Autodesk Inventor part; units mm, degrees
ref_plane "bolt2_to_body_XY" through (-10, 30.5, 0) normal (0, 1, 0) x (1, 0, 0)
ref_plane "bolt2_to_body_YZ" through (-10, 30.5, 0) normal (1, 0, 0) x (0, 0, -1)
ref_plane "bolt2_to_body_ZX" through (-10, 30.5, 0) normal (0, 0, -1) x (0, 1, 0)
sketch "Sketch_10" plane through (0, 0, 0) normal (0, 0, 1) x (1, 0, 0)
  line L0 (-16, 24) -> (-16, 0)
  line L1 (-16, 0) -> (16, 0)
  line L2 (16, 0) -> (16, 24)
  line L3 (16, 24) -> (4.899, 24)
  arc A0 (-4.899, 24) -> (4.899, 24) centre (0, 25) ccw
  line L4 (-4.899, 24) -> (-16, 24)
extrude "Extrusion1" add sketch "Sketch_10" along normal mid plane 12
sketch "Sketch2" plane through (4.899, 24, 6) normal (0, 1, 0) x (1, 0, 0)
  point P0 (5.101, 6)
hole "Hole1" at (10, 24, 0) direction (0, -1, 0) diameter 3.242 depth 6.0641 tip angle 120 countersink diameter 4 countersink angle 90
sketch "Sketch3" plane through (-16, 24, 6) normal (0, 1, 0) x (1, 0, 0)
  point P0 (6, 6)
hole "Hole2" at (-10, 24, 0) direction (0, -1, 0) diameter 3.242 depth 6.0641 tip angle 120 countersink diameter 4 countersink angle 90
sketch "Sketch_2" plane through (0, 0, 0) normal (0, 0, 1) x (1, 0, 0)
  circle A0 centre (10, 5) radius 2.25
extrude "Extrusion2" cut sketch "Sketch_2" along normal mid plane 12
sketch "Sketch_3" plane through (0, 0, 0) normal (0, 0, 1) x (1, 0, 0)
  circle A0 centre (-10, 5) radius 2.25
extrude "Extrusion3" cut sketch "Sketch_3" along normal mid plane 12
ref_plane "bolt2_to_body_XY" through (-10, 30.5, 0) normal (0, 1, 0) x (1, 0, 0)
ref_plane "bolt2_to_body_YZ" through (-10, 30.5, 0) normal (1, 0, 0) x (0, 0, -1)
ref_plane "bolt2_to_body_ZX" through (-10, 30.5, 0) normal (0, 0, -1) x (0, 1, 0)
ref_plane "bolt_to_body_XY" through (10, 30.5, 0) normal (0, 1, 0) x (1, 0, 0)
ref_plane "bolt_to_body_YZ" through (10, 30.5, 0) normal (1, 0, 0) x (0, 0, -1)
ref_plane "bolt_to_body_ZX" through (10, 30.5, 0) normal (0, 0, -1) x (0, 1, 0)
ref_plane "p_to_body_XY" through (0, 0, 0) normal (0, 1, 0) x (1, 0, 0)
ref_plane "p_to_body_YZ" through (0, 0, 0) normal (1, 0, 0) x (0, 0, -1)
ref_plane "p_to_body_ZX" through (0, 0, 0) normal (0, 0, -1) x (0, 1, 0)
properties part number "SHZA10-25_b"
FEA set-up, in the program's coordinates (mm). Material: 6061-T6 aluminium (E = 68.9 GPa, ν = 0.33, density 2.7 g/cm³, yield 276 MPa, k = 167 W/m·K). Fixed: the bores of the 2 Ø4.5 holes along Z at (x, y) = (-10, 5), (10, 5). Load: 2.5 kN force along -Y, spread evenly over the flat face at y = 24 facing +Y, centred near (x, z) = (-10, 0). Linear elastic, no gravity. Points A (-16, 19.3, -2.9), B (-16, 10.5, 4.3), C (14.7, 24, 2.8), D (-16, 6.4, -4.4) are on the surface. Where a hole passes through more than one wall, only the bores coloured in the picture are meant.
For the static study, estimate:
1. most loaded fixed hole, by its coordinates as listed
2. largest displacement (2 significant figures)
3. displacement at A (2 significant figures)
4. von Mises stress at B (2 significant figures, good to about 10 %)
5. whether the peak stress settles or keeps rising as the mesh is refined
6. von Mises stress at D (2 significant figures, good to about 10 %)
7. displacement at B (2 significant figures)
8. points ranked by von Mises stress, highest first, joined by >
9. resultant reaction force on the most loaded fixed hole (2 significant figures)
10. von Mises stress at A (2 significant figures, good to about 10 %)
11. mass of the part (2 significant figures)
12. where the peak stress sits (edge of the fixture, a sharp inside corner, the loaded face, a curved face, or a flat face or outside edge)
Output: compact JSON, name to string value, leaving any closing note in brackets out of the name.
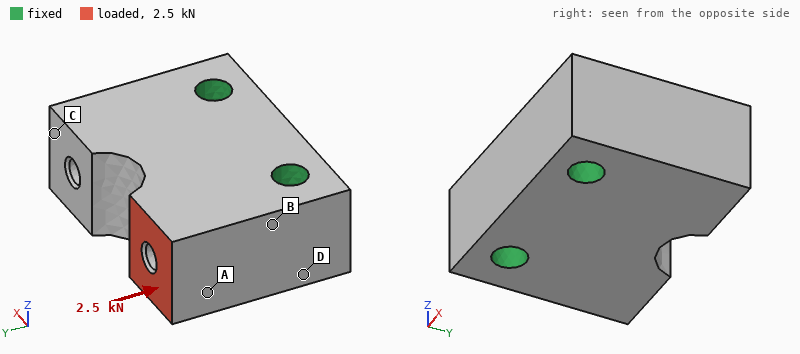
{"most loaded fixed hole, by its coordinates as listed": "(-10, 5)", "largest displacement": "7.5 µm", "displacement at A": "5.6 µm", "von Mises stress at B": "17 MPa", "whether the peak stress settles or keeps rising as the mesh is refined": "keeps rising", "von Mises stress at D": "10 MPa", "displacement at B": "2.5 µm", "points ranked by von Mises stress, highest first, joined by >": "A > B > D > C", "resultant reaction force on the most loaded fixed hole": "2.4 kN", "von Mises stress at A": "22 MPa", "mass of the part": "23 g", "where the peak stress sits": "edge of the fixture"}
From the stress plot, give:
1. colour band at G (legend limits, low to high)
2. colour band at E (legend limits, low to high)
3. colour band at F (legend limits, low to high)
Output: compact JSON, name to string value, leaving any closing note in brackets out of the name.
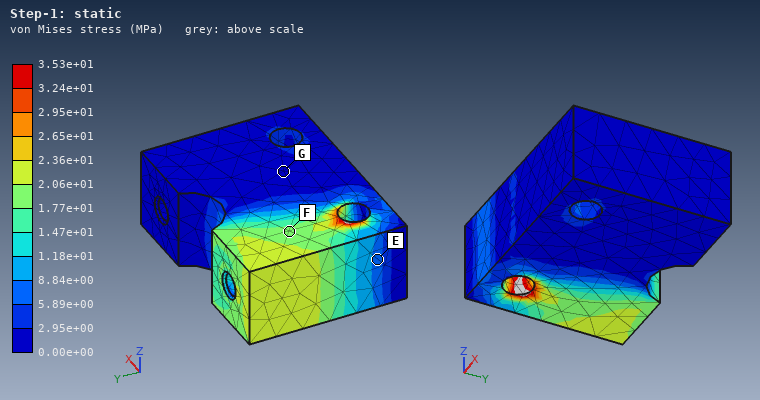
{"colour band at G": "0.00e+00 to 2.95e+00 MPa", "colour band at E": "5.89e+00 to 8.84e+00 MPa", "colour band at F": "1.77e+01 to 2.06e+01 MPa"}
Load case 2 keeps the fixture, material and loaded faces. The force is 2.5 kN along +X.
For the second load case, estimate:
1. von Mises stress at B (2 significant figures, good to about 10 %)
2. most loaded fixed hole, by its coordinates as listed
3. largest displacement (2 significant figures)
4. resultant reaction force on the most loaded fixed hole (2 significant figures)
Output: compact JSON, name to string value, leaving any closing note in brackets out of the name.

{"von Mises stress at B": "29 MPa", "most loaded fixed hole, by its coordinates as listed": "(10, 5)", "largest displacement": "23 µm", "resultant reaction force on the most loaded fixed hole": "2.6 kN"}
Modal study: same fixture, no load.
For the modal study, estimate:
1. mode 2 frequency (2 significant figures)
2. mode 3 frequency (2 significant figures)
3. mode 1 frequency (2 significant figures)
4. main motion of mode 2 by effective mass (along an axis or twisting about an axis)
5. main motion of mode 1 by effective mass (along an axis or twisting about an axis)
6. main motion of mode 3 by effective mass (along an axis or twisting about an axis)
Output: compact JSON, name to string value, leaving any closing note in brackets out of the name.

{"mode 2 frequency": "31 kHz", "mode 3 frequency": "34 kHz", "mode 1 frequency": "22 kHz", "main motion of mode 2 by effective mass": "twisting about Y", "main motion of mode 1 by effective mass": "along Z", "main motion of mode 3 by effective mass": "along X"}
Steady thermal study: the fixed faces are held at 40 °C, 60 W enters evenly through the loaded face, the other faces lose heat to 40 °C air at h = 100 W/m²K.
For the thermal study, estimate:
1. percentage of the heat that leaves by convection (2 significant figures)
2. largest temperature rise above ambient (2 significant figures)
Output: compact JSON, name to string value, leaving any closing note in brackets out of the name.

{"percentage of the heat that leaves by convection": "3.4 %", "largest temperature rise above ambient": "38 K"}
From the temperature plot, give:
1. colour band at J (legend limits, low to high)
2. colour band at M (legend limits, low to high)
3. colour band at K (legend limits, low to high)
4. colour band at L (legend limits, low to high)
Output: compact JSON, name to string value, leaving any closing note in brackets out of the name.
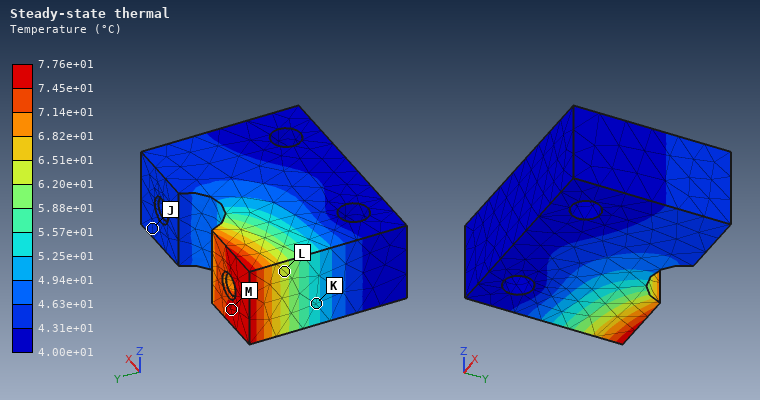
{"colour band at J": "4.31e+01 to 4.63e+01 °C", "colour band at M": "7.45e+01 to 7.76e+01 °C", "colour band at K": "5.25e+01 to 5.57e+01 °C", "colour band at L": "6.20e+01 to 6.51e+01 °C"}
